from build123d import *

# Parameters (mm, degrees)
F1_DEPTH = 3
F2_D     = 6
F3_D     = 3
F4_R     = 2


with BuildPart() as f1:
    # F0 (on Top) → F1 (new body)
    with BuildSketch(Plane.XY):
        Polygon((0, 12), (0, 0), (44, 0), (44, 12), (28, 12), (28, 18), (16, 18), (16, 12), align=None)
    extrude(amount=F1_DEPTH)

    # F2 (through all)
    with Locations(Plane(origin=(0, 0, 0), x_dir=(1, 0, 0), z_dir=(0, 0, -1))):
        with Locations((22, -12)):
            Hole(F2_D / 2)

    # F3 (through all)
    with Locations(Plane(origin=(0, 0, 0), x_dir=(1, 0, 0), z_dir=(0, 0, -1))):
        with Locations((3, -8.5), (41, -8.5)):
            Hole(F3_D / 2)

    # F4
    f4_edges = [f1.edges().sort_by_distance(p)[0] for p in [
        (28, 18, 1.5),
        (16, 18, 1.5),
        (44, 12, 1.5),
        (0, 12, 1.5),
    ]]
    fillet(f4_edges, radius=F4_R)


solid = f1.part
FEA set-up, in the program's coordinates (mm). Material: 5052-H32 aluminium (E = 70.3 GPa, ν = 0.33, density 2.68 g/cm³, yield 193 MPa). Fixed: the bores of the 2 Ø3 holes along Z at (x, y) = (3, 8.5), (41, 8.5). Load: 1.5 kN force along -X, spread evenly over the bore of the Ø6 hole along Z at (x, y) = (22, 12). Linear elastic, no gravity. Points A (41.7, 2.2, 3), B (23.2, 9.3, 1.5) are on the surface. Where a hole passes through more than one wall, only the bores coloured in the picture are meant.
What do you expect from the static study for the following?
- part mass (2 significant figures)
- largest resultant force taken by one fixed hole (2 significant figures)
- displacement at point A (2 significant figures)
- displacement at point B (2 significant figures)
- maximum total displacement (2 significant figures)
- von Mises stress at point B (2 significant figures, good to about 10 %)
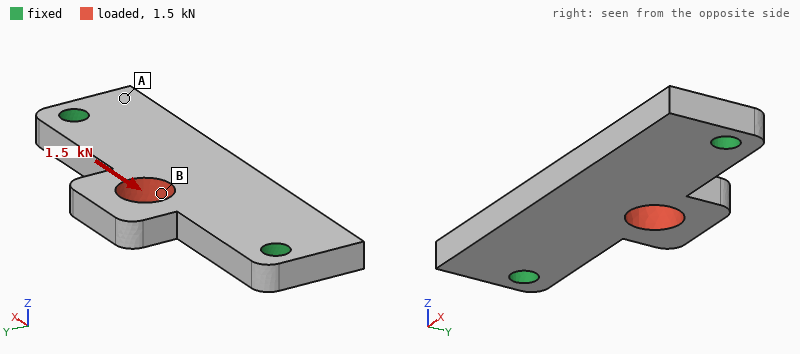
4.5 g
770 N
3.7 µm
8.3 µm
22 µm
45 MPa
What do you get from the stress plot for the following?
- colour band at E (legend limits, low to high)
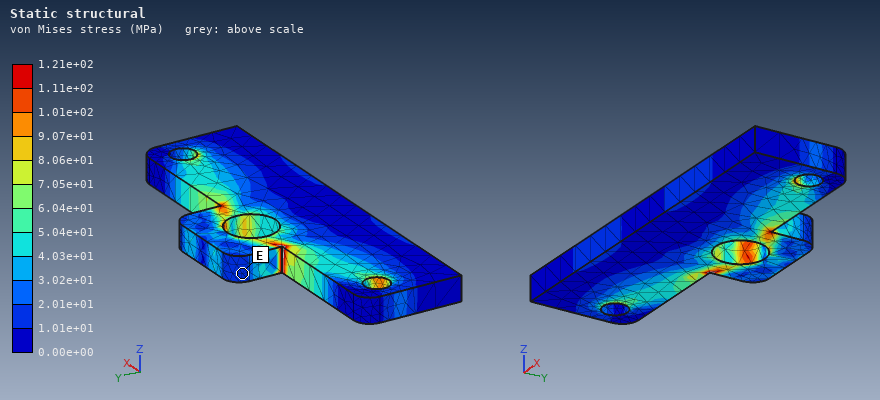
1.01e+01 to 2.01e+01 MPa
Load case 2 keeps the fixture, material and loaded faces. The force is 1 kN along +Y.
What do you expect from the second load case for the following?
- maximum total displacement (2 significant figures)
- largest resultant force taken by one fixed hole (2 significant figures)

26 µm
600 N
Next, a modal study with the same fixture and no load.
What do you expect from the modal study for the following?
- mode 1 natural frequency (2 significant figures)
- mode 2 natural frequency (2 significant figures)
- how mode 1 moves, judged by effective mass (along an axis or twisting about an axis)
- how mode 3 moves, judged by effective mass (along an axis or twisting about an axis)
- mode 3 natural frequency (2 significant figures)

9100 Hz
12 kHz
along Z
along Y
21 kHz
